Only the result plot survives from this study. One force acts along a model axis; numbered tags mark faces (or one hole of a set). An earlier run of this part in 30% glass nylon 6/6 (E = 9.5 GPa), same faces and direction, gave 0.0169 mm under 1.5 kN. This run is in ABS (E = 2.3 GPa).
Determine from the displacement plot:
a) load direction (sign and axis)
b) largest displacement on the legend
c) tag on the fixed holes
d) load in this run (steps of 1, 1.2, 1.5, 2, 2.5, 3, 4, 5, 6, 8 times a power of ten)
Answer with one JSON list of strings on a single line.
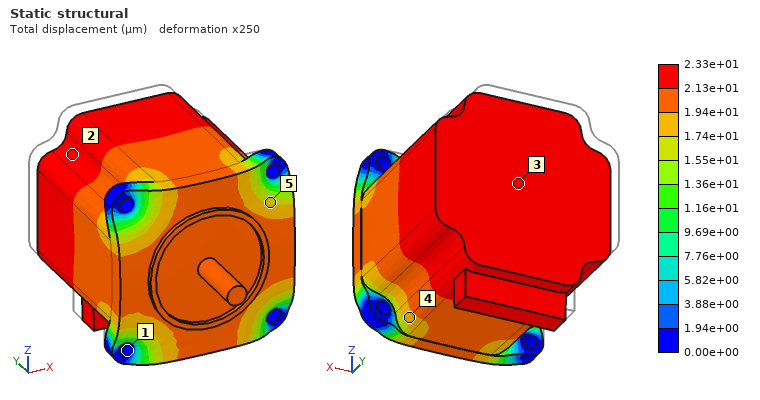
["-Y", "2.33e+01 µm", "1", "500 N"]
